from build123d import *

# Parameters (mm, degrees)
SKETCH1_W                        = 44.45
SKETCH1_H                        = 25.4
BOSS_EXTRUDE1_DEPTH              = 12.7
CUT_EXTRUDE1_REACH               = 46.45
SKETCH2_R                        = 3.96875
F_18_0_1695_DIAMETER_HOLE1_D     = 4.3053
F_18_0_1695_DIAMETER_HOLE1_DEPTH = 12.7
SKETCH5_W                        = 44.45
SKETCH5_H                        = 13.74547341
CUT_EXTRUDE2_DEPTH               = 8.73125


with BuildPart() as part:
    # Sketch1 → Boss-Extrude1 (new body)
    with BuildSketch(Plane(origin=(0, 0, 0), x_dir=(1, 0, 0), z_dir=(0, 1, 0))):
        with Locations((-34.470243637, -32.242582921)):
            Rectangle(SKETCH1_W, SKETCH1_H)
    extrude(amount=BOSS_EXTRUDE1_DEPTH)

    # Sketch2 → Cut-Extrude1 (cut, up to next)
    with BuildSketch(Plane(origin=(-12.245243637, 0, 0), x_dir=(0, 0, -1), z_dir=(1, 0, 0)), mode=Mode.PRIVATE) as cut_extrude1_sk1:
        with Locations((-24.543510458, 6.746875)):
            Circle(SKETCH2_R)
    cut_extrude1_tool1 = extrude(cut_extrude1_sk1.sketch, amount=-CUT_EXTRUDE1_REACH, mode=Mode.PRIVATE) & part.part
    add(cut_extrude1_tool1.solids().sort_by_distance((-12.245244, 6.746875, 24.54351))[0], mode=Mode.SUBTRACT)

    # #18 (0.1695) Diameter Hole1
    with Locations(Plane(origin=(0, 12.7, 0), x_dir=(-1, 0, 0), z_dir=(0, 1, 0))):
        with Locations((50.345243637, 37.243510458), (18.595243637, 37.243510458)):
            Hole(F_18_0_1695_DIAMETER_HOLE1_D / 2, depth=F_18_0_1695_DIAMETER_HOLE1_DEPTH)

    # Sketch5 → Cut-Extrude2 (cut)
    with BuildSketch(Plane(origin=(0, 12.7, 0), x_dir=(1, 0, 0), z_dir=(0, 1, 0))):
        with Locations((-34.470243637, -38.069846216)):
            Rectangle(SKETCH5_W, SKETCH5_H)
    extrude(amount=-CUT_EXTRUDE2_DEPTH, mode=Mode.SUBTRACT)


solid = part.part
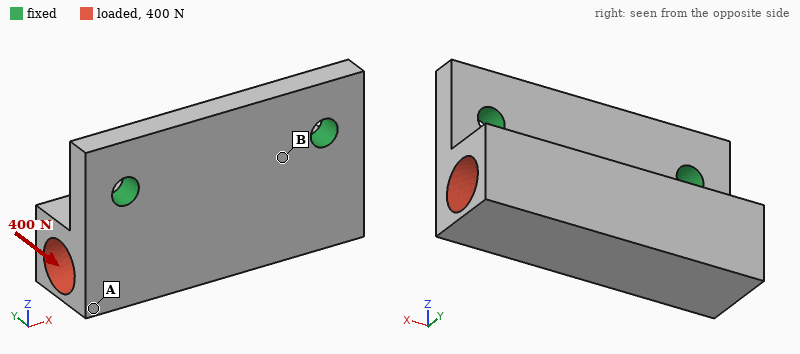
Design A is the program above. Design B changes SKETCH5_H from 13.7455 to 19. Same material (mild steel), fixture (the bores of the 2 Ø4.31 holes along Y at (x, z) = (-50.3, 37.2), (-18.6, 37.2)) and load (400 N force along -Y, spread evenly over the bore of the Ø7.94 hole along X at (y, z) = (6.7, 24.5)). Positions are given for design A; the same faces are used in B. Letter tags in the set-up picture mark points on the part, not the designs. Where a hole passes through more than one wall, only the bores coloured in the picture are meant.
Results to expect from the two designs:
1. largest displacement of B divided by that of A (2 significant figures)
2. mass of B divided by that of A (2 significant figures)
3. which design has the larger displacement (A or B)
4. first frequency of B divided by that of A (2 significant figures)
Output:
1.1
0.85
B
0.94
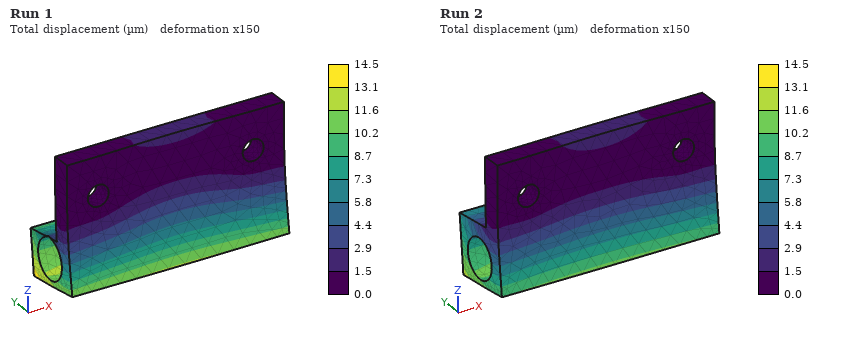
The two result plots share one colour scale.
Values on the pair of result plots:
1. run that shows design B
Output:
Run 1
